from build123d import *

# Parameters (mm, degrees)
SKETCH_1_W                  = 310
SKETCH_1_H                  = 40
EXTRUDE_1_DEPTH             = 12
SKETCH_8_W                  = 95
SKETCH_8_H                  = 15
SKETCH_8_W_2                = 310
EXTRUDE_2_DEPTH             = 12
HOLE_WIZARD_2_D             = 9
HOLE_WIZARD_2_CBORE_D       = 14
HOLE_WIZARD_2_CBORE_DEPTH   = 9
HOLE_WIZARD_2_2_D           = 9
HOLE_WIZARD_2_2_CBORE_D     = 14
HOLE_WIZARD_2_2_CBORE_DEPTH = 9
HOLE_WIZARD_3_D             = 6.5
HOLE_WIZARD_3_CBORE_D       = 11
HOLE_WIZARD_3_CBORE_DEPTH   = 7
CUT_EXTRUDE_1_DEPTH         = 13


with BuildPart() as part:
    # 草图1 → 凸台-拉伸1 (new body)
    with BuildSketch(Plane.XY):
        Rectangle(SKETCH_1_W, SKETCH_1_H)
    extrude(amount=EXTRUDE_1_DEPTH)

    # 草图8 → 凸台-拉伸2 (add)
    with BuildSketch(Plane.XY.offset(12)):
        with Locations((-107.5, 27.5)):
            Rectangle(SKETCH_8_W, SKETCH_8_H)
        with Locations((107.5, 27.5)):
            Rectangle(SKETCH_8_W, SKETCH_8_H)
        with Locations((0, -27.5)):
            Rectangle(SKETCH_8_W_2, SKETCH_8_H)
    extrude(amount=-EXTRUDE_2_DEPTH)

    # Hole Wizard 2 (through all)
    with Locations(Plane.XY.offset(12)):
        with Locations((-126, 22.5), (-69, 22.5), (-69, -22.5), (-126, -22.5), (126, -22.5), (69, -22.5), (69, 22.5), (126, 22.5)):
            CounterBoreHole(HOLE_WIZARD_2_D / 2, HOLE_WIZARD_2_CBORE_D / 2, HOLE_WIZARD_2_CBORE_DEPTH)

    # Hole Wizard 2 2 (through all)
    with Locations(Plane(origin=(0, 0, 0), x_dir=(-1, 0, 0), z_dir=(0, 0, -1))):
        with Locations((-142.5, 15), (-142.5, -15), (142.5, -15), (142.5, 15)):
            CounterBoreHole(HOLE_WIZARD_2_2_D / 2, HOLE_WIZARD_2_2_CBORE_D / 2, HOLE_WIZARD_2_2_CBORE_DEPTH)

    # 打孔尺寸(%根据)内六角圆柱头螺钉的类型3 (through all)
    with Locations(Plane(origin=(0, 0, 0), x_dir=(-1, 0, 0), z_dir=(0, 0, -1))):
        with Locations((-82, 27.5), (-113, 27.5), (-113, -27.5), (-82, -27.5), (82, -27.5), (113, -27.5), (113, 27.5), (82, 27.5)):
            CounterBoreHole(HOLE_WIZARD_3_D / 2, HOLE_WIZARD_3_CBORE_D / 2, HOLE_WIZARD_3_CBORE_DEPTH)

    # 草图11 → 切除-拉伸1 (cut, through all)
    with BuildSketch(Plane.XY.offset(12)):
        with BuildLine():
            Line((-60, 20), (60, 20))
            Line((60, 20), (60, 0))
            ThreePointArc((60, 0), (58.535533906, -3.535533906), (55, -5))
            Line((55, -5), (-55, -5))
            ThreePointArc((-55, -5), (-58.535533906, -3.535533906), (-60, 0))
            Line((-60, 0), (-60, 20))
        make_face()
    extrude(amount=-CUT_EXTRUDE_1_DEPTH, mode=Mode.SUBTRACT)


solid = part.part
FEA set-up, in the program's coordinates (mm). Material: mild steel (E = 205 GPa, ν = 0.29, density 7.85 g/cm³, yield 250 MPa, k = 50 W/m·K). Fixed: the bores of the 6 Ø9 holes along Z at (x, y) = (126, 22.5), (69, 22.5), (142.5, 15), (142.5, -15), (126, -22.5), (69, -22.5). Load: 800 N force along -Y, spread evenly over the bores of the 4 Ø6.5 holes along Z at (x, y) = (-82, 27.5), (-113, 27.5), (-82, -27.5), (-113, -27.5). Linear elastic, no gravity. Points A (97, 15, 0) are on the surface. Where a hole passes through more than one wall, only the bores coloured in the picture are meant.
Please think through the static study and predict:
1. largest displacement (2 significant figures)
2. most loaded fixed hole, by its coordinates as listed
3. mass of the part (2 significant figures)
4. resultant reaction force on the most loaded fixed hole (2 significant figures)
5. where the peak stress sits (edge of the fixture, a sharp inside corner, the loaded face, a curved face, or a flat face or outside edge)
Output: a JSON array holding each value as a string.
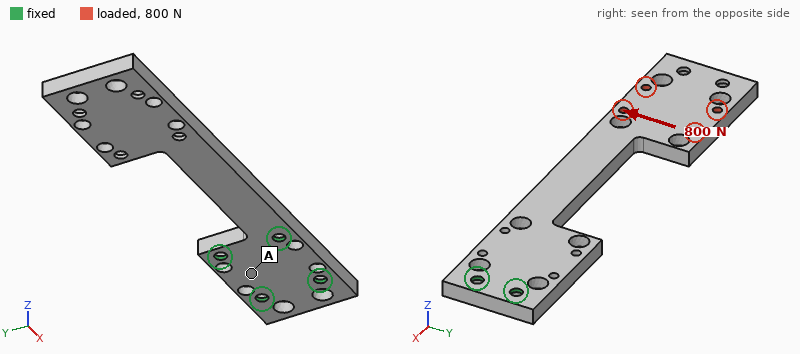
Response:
["0.41 mm", "(69, -22.5)", "1.4 kg", "2.2 kN", "edge of the fixture"]
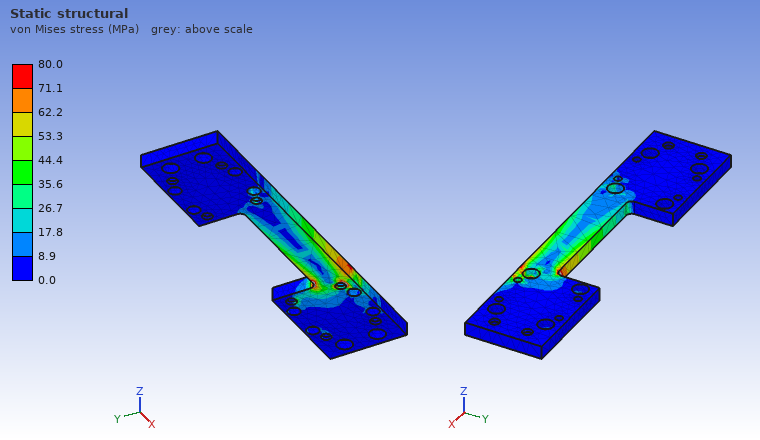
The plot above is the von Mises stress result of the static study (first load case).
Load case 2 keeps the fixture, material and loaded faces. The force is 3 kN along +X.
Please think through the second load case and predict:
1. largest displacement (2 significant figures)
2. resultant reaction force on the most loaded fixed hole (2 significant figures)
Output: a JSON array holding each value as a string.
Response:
["0.42 mm", "710 N"]
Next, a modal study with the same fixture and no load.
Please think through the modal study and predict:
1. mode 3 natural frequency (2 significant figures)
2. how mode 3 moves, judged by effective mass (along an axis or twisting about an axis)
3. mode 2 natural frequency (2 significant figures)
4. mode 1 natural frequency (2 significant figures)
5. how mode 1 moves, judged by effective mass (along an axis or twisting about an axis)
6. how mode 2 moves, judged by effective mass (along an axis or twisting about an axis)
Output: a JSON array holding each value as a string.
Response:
["840 Hz", "twisting about X", "330 Hz", "130 Hz", "along Z", "along Y"]
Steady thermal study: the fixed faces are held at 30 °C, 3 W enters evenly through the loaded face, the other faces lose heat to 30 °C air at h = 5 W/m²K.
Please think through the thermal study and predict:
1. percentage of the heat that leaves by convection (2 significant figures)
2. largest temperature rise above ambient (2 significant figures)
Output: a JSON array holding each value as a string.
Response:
["55 %", "15 K"]
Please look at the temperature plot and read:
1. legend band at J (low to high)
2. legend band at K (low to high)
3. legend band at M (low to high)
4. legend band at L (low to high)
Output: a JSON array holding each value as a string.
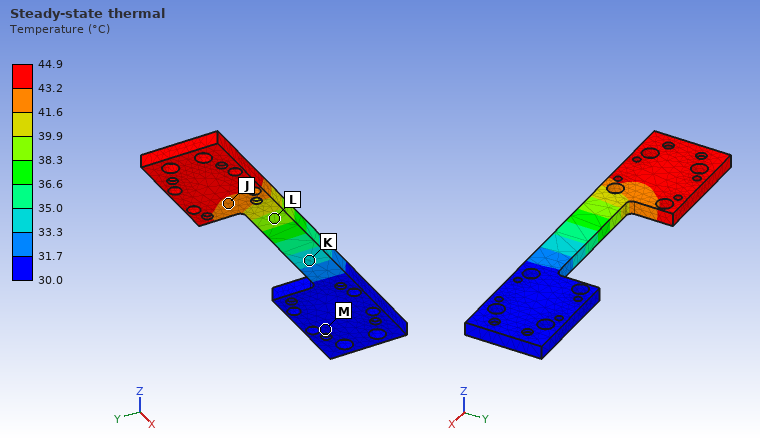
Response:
["41.6 to 43.2 °C", "33.3 to 35.0 °C", "30.0 to 31.7 °C", "38.3 to 39.9 °C"]
